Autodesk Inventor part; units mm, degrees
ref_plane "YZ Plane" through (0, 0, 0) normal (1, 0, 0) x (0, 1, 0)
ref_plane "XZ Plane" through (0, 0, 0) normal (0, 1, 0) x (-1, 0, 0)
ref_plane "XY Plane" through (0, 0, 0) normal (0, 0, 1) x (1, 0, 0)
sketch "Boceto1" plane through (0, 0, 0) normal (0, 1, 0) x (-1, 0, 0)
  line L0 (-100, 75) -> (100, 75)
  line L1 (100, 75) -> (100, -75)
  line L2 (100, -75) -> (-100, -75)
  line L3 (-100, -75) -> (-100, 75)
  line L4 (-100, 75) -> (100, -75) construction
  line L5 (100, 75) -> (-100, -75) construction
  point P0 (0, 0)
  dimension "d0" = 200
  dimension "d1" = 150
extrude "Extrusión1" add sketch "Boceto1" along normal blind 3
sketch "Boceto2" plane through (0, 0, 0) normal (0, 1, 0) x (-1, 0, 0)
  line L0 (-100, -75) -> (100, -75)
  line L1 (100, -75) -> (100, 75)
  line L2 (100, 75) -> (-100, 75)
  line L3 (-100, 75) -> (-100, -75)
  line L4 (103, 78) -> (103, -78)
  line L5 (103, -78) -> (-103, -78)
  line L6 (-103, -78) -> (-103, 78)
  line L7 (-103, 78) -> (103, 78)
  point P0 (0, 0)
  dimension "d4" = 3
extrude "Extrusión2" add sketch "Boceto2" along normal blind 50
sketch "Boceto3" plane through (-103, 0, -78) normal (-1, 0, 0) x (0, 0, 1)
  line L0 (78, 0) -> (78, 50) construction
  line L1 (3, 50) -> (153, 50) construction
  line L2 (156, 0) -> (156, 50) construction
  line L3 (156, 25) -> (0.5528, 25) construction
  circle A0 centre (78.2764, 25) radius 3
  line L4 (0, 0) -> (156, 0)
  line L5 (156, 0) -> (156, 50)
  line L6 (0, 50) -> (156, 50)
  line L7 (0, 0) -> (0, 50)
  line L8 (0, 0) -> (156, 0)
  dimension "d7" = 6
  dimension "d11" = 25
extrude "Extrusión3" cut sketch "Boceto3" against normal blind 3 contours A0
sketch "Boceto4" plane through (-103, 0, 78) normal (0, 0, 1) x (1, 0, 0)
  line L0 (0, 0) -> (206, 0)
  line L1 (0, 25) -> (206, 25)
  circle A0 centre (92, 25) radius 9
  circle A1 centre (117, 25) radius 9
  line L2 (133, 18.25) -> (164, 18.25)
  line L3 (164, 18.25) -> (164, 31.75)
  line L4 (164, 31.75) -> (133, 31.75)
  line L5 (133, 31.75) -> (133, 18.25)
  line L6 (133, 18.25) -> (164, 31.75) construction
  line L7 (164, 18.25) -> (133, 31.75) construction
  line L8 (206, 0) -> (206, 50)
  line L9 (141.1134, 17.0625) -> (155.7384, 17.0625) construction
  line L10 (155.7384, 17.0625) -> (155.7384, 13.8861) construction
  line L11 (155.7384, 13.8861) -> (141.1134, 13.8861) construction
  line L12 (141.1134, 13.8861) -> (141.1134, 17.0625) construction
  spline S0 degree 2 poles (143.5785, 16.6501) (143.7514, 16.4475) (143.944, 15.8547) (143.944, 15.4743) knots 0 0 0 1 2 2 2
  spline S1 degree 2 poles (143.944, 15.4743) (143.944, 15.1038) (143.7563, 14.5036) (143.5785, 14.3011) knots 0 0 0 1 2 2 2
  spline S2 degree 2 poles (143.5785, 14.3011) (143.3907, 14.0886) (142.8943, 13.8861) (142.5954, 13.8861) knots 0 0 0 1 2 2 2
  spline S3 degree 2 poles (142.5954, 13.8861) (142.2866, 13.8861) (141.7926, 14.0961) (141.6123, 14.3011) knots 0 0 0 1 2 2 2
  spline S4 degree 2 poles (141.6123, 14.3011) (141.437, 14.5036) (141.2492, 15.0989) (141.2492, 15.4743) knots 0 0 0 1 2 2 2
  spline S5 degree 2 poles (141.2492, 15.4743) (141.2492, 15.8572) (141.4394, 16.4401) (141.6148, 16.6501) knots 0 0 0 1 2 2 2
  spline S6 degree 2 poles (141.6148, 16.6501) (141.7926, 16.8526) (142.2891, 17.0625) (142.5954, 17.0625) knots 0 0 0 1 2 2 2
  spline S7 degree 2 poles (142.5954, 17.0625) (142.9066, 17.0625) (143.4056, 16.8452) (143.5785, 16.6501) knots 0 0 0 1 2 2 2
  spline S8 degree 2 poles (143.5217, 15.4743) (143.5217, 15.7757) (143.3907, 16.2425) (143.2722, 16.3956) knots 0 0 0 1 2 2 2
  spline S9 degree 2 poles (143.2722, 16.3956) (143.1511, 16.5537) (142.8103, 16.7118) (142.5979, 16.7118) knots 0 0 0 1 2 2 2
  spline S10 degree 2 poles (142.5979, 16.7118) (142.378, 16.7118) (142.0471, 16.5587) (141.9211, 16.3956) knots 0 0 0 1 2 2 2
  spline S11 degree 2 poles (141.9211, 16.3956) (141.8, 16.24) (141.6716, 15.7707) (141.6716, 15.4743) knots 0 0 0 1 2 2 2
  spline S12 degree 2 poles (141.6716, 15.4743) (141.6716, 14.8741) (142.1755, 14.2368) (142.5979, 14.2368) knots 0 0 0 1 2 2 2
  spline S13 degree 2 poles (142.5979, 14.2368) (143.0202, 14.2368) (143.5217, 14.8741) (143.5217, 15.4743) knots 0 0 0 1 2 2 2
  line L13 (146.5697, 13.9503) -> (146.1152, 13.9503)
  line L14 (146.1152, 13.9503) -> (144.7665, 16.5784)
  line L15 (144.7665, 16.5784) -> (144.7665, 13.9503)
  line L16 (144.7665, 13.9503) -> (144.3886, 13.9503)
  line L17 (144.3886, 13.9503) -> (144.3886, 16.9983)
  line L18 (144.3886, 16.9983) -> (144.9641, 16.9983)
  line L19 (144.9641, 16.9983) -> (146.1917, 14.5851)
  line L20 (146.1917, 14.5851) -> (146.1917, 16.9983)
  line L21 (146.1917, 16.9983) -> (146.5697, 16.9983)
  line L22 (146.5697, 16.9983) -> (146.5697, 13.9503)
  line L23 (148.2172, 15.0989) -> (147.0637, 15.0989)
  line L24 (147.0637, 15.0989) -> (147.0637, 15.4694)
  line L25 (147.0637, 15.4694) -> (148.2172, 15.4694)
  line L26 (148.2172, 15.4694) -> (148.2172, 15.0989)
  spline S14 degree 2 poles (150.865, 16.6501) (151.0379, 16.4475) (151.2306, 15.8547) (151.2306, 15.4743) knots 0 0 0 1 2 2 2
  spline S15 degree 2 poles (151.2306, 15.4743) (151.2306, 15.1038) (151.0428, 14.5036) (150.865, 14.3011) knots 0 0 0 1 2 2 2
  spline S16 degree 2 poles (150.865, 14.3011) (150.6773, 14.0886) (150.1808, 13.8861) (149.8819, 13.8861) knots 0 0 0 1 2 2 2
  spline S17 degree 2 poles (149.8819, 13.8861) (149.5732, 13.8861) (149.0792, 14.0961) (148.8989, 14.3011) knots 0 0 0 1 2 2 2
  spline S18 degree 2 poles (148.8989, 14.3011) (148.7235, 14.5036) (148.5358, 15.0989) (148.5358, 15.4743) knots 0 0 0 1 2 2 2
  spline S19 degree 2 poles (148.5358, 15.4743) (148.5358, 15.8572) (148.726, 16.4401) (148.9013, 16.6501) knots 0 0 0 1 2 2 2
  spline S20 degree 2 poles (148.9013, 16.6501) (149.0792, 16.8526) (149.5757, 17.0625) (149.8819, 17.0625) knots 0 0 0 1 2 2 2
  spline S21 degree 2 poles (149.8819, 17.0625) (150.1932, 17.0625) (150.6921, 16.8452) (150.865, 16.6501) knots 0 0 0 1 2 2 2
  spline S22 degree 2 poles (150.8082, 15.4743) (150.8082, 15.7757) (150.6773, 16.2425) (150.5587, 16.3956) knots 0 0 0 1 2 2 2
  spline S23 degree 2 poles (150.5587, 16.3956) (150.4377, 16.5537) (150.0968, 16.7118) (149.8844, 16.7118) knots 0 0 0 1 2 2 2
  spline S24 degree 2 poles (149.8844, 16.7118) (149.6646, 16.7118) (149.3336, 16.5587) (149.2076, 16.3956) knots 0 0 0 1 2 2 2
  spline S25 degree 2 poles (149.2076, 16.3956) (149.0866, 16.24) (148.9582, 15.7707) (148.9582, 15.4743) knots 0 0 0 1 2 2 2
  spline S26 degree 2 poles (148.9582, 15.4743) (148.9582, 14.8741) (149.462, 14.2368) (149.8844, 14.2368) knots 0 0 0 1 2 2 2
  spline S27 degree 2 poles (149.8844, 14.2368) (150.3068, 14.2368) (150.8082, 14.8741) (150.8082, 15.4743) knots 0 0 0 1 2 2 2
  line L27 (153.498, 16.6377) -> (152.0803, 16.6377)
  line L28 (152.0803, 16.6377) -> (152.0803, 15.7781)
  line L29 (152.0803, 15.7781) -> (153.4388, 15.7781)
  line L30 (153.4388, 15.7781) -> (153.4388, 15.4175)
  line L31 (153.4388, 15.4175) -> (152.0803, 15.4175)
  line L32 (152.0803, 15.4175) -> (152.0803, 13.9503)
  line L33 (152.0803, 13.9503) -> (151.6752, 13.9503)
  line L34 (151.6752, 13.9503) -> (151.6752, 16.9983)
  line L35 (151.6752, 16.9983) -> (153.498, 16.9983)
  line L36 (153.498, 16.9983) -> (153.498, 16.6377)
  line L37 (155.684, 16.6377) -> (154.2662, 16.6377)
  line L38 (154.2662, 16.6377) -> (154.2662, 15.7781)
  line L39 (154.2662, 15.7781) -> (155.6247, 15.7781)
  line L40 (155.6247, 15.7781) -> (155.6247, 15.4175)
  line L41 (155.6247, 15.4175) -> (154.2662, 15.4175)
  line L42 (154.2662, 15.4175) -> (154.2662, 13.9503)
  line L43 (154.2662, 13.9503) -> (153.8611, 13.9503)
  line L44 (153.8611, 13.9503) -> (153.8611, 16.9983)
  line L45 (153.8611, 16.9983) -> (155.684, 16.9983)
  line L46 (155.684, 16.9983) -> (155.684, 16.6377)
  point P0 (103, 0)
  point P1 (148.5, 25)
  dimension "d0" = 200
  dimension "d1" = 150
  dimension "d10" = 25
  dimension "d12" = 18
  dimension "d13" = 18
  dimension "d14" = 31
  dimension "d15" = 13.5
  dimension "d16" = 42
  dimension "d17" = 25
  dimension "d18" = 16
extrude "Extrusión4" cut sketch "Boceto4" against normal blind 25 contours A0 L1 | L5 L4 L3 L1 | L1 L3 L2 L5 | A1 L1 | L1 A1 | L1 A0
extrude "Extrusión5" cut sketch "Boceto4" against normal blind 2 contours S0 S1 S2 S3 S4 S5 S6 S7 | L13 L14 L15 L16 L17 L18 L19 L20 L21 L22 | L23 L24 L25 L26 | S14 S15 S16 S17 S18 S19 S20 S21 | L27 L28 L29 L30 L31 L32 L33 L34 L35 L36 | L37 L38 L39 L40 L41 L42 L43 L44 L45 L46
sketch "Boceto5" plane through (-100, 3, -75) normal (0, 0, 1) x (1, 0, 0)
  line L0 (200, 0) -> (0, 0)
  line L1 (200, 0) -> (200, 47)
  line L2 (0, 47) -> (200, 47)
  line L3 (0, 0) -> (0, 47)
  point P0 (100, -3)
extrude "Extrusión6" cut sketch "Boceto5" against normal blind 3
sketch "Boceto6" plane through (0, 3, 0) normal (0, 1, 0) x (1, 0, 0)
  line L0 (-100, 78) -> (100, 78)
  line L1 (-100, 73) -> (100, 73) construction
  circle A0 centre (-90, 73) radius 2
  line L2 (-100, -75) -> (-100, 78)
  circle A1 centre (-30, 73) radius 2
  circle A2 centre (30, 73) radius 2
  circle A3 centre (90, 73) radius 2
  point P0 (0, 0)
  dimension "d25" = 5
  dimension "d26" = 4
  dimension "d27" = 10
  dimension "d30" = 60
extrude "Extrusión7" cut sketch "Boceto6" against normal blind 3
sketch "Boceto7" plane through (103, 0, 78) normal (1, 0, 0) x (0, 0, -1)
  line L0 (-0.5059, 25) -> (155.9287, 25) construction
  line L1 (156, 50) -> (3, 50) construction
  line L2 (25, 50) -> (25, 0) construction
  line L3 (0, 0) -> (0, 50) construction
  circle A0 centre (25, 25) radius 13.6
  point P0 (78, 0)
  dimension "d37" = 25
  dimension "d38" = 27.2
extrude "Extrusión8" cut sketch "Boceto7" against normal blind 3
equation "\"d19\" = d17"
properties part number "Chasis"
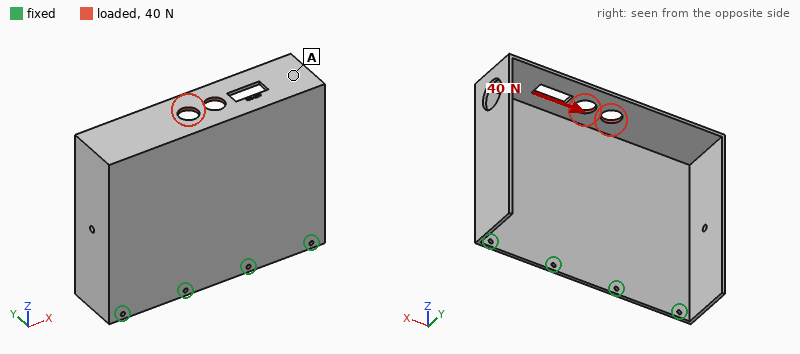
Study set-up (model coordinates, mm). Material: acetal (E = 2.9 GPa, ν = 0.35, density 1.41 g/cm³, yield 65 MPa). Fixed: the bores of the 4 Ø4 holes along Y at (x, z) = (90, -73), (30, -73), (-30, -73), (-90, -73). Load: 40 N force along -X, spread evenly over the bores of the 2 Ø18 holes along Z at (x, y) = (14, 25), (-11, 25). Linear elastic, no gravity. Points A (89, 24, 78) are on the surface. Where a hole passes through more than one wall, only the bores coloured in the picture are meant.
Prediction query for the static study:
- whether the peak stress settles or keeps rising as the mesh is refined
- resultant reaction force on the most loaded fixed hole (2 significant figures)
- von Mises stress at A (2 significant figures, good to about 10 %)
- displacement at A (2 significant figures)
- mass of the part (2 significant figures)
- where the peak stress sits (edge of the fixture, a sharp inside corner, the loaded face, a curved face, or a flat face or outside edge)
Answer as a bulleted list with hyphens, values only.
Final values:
- keeps rising
- 32 N
- 0.49 MPa
- 2.0 mm
- 230 g
- edge of the fixture
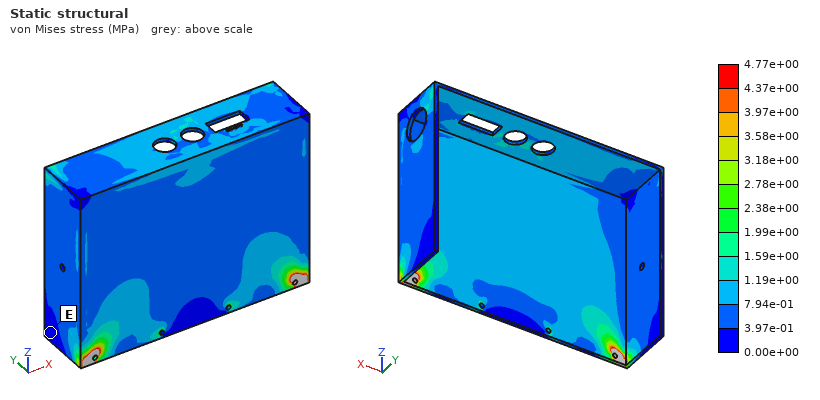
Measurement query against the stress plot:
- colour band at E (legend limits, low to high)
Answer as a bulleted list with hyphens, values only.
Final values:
- 0.00e+00 to 3.97e-01 MPa
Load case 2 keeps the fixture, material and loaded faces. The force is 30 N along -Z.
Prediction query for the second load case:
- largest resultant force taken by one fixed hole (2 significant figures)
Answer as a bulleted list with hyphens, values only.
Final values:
- 9.4 N
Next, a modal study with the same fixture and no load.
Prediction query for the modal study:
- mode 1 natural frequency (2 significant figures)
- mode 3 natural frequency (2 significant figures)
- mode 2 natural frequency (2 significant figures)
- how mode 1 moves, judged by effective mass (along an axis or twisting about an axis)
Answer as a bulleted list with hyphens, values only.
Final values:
- 28 Hz
- 180 Hz
- 45 Hz
- along Y
